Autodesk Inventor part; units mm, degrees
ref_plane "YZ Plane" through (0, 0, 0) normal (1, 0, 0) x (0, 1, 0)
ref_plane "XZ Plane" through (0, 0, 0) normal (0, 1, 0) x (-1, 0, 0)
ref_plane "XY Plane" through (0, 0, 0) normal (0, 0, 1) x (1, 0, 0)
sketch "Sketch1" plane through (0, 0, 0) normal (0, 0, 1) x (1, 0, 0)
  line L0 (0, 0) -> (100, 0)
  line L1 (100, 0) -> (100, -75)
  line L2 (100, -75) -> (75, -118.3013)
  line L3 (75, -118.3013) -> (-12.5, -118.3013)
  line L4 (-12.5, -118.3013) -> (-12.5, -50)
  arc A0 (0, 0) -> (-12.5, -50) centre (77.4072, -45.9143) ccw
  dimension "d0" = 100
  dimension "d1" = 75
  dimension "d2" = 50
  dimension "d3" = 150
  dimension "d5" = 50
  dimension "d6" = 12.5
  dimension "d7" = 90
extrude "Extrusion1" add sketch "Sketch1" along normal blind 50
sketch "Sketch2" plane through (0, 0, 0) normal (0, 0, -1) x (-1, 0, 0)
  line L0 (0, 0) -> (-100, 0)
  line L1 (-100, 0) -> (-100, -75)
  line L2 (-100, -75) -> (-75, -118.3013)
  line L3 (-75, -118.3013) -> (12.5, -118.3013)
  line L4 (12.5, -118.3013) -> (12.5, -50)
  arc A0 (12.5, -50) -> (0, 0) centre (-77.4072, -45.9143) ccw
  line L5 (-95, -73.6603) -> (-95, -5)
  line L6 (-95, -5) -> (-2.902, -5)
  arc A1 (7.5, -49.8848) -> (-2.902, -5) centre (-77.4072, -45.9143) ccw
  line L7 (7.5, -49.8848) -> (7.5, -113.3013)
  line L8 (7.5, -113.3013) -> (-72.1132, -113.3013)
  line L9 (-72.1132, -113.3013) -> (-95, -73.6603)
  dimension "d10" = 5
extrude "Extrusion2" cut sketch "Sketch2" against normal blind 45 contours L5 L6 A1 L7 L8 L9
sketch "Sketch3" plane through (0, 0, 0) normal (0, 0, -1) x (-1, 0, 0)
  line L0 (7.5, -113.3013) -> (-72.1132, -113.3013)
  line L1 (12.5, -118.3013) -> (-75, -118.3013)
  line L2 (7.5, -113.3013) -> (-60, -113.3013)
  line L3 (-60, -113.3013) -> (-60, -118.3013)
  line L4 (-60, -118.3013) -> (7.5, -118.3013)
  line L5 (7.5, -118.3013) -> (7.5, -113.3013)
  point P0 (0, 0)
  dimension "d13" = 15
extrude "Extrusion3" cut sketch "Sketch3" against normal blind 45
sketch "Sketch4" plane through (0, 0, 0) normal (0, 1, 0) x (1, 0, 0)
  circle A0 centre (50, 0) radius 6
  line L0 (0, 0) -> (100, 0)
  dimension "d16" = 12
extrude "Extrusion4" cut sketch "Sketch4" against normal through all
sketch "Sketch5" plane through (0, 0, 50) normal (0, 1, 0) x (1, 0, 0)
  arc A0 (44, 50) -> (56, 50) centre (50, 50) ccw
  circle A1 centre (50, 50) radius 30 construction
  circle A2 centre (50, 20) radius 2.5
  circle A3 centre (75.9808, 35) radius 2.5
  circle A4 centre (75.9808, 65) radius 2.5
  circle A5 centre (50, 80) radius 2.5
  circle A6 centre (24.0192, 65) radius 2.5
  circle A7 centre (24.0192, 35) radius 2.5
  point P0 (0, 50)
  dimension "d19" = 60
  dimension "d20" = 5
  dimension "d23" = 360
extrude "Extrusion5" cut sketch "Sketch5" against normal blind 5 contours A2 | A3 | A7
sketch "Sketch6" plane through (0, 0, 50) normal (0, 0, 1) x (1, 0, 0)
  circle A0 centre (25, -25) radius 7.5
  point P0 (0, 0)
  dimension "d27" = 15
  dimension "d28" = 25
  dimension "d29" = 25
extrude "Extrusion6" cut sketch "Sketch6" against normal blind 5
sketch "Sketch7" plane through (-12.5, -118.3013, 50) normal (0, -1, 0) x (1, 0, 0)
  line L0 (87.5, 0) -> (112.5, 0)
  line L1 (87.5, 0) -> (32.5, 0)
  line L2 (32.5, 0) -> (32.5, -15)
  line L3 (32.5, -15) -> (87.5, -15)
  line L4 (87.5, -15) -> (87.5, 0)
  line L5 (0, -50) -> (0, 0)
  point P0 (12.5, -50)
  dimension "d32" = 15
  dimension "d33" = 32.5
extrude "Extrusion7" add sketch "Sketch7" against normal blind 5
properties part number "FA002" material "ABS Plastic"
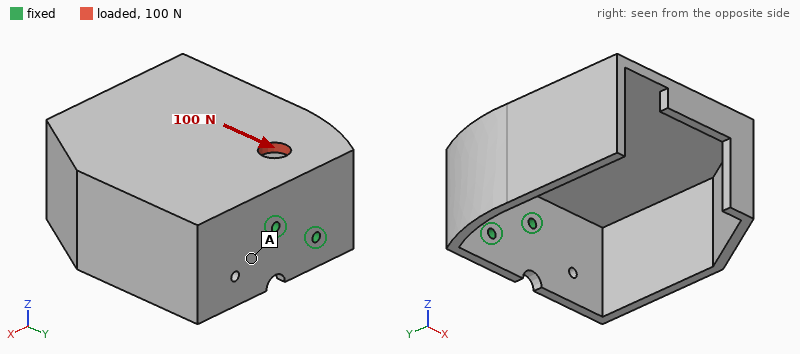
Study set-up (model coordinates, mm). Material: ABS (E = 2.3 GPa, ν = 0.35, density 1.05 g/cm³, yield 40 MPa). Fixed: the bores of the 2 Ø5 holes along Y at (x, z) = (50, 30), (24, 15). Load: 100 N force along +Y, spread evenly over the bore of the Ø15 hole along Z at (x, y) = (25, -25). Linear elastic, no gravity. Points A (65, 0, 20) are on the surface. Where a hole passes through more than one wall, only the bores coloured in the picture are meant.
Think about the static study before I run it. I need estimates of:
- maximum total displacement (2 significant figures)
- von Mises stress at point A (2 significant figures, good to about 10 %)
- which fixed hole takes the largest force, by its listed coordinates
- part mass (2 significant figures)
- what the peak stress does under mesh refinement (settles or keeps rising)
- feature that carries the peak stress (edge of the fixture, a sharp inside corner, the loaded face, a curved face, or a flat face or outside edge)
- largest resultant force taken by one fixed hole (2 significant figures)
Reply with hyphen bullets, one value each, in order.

- 1.8 mm
- 1.1 MPa
- (50, 30)
- 150 g
- keeps rising
- edge of the fixture
- 57 N
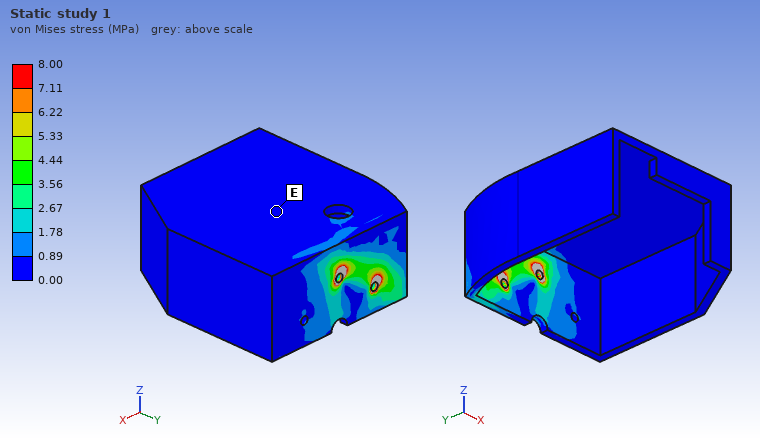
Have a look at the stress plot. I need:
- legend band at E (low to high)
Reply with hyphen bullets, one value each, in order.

- 0.00 to 0.89 MPa
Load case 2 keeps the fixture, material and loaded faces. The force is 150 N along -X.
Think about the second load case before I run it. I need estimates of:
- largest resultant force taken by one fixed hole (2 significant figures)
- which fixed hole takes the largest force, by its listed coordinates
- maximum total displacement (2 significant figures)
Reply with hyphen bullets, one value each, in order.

- 190 N
- (50, 30)
- 1.7 mm
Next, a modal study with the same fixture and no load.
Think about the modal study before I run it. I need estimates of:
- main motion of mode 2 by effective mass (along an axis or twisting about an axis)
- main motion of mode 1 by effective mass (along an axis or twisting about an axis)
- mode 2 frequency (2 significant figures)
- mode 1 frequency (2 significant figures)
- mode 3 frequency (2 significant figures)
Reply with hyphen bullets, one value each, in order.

- along X
- along Z
- 100 Hz
- 74 Hz
- 230 Hz
